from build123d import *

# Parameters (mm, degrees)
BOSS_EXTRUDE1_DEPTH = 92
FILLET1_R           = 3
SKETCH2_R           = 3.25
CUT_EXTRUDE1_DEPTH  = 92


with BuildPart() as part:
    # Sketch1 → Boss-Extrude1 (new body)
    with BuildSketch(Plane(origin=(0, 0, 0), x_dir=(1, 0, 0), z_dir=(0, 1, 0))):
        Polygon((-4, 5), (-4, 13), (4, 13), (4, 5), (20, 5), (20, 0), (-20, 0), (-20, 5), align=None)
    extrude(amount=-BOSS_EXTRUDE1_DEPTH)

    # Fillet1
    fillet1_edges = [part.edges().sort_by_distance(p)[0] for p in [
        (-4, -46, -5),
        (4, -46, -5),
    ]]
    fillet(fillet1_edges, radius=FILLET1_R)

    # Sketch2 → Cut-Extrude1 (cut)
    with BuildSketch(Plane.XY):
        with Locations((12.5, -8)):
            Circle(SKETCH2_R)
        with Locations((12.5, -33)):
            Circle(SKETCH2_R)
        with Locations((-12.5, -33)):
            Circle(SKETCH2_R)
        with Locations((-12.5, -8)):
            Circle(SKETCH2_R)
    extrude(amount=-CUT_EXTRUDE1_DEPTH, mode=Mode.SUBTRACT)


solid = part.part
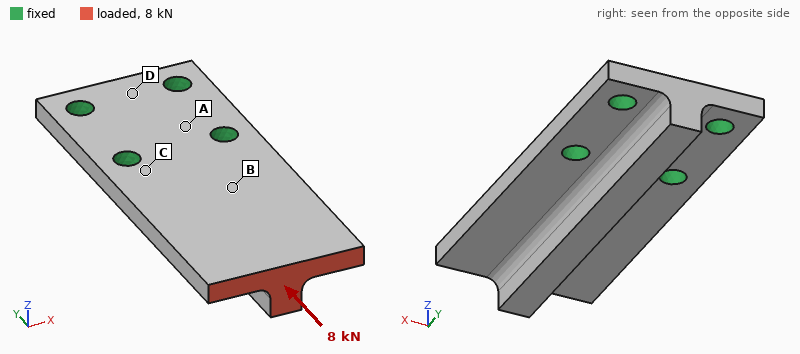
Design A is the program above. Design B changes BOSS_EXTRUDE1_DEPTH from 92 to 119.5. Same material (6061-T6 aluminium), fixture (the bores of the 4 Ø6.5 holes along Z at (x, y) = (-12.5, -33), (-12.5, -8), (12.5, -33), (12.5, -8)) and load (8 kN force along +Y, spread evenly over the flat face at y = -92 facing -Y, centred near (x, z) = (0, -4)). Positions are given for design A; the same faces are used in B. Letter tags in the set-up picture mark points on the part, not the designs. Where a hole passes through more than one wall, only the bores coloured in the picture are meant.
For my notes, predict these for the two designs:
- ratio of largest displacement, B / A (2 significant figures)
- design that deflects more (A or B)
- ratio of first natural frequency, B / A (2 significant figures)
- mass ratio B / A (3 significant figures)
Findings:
1.4
B
0.50
1.31
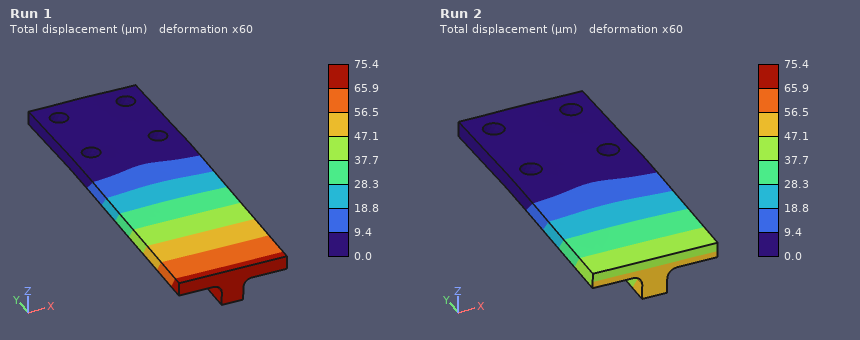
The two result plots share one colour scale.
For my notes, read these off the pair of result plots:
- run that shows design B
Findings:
Run 1
